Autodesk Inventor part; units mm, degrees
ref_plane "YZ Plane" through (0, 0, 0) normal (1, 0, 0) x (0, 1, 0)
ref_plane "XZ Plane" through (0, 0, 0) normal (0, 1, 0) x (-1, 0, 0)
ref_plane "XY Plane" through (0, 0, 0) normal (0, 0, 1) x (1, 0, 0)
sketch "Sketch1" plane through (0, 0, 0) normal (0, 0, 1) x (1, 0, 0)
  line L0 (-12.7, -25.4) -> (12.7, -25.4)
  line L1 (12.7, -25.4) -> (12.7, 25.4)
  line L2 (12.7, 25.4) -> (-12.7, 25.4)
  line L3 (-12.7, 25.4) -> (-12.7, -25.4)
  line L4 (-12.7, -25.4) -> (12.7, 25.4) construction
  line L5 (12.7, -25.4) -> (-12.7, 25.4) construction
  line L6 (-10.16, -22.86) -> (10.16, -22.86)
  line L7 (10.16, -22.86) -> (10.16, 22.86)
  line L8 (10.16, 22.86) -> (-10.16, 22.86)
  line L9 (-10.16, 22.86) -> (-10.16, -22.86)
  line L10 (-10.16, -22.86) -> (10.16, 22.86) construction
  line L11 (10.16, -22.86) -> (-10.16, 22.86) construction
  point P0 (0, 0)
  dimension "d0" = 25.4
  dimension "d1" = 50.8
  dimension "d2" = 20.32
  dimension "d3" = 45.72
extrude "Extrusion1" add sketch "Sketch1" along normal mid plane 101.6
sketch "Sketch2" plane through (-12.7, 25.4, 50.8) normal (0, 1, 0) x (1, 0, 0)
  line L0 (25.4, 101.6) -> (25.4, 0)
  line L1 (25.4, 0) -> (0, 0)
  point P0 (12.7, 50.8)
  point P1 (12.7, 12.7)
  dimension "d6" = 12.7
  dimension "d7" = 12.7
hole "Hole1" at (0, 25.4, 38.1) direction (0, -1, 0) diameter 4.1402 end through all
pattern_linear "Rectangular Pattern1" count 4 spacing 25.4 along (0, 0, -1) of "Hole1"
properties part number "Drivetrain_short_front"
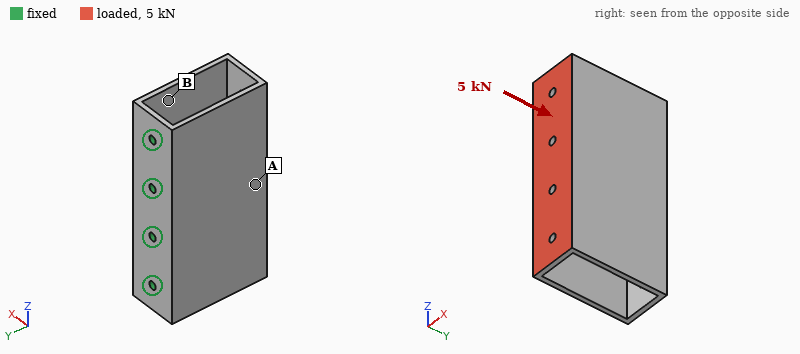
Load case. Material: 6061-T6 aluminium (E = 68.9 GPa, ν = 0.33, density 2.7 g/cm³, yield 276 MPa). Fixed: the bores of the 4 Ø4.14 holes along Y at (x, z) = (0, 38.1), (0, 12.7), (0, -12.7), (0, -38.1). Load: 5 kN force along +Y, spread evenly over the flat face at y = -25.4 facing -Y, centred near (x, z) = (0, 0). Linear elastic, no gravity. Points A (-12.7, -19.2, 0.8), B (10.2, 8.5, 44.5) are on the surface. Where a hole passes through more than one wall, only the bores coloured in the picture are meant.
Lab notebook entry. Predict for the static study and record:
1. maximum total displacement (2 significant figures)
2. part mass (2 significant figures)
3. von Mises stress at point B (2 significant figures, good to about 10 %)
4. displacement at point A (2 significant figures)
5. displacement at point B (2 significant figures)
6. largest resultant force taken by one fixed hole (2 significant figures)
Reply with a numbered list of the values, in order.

1. 0.15 mm
2. 98 g
3. 44 MPa
4. 0.086 mm
5. 0.12 mm
6. 1.3 kN
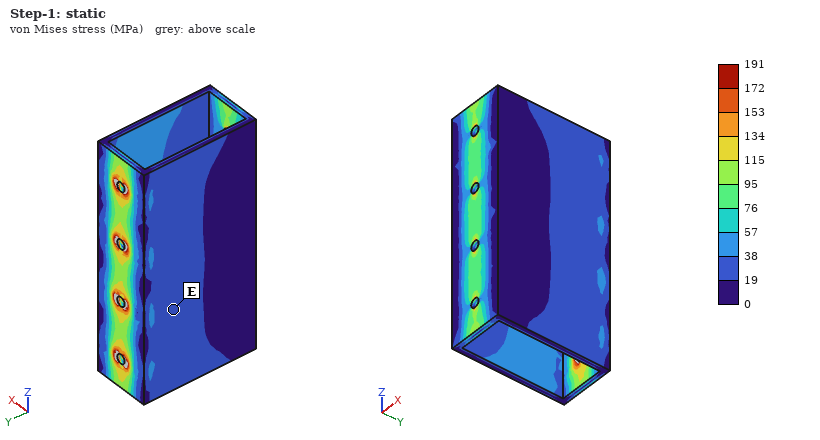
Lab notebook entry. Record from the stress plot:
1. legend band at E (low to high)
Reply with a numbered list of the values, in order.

1. 19 to 38 MPa
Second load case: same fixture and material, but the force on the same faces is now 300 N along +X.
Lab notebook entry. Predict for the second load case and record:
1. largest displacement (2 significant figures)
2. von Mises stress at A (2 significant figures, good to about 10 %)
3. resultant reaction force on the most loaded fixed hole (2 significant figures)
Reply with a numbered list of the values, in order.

1. 0.43 mm
2. 22 MPa
3. 86 N
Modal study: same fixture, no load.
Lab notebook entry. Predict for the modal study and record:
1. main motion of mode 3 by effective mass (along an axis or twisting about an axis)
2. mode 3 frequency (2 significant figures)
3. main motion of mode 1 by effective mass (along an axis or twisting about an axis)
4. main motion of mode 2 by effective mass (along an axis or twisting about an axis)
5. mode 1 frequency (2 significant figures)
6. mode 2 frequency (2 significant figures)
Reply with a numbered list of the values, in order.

1. along Z
2. 2800 Hz
3. along X
4. twisting about Y
5. 670 Hz
6. 2200 Hz
